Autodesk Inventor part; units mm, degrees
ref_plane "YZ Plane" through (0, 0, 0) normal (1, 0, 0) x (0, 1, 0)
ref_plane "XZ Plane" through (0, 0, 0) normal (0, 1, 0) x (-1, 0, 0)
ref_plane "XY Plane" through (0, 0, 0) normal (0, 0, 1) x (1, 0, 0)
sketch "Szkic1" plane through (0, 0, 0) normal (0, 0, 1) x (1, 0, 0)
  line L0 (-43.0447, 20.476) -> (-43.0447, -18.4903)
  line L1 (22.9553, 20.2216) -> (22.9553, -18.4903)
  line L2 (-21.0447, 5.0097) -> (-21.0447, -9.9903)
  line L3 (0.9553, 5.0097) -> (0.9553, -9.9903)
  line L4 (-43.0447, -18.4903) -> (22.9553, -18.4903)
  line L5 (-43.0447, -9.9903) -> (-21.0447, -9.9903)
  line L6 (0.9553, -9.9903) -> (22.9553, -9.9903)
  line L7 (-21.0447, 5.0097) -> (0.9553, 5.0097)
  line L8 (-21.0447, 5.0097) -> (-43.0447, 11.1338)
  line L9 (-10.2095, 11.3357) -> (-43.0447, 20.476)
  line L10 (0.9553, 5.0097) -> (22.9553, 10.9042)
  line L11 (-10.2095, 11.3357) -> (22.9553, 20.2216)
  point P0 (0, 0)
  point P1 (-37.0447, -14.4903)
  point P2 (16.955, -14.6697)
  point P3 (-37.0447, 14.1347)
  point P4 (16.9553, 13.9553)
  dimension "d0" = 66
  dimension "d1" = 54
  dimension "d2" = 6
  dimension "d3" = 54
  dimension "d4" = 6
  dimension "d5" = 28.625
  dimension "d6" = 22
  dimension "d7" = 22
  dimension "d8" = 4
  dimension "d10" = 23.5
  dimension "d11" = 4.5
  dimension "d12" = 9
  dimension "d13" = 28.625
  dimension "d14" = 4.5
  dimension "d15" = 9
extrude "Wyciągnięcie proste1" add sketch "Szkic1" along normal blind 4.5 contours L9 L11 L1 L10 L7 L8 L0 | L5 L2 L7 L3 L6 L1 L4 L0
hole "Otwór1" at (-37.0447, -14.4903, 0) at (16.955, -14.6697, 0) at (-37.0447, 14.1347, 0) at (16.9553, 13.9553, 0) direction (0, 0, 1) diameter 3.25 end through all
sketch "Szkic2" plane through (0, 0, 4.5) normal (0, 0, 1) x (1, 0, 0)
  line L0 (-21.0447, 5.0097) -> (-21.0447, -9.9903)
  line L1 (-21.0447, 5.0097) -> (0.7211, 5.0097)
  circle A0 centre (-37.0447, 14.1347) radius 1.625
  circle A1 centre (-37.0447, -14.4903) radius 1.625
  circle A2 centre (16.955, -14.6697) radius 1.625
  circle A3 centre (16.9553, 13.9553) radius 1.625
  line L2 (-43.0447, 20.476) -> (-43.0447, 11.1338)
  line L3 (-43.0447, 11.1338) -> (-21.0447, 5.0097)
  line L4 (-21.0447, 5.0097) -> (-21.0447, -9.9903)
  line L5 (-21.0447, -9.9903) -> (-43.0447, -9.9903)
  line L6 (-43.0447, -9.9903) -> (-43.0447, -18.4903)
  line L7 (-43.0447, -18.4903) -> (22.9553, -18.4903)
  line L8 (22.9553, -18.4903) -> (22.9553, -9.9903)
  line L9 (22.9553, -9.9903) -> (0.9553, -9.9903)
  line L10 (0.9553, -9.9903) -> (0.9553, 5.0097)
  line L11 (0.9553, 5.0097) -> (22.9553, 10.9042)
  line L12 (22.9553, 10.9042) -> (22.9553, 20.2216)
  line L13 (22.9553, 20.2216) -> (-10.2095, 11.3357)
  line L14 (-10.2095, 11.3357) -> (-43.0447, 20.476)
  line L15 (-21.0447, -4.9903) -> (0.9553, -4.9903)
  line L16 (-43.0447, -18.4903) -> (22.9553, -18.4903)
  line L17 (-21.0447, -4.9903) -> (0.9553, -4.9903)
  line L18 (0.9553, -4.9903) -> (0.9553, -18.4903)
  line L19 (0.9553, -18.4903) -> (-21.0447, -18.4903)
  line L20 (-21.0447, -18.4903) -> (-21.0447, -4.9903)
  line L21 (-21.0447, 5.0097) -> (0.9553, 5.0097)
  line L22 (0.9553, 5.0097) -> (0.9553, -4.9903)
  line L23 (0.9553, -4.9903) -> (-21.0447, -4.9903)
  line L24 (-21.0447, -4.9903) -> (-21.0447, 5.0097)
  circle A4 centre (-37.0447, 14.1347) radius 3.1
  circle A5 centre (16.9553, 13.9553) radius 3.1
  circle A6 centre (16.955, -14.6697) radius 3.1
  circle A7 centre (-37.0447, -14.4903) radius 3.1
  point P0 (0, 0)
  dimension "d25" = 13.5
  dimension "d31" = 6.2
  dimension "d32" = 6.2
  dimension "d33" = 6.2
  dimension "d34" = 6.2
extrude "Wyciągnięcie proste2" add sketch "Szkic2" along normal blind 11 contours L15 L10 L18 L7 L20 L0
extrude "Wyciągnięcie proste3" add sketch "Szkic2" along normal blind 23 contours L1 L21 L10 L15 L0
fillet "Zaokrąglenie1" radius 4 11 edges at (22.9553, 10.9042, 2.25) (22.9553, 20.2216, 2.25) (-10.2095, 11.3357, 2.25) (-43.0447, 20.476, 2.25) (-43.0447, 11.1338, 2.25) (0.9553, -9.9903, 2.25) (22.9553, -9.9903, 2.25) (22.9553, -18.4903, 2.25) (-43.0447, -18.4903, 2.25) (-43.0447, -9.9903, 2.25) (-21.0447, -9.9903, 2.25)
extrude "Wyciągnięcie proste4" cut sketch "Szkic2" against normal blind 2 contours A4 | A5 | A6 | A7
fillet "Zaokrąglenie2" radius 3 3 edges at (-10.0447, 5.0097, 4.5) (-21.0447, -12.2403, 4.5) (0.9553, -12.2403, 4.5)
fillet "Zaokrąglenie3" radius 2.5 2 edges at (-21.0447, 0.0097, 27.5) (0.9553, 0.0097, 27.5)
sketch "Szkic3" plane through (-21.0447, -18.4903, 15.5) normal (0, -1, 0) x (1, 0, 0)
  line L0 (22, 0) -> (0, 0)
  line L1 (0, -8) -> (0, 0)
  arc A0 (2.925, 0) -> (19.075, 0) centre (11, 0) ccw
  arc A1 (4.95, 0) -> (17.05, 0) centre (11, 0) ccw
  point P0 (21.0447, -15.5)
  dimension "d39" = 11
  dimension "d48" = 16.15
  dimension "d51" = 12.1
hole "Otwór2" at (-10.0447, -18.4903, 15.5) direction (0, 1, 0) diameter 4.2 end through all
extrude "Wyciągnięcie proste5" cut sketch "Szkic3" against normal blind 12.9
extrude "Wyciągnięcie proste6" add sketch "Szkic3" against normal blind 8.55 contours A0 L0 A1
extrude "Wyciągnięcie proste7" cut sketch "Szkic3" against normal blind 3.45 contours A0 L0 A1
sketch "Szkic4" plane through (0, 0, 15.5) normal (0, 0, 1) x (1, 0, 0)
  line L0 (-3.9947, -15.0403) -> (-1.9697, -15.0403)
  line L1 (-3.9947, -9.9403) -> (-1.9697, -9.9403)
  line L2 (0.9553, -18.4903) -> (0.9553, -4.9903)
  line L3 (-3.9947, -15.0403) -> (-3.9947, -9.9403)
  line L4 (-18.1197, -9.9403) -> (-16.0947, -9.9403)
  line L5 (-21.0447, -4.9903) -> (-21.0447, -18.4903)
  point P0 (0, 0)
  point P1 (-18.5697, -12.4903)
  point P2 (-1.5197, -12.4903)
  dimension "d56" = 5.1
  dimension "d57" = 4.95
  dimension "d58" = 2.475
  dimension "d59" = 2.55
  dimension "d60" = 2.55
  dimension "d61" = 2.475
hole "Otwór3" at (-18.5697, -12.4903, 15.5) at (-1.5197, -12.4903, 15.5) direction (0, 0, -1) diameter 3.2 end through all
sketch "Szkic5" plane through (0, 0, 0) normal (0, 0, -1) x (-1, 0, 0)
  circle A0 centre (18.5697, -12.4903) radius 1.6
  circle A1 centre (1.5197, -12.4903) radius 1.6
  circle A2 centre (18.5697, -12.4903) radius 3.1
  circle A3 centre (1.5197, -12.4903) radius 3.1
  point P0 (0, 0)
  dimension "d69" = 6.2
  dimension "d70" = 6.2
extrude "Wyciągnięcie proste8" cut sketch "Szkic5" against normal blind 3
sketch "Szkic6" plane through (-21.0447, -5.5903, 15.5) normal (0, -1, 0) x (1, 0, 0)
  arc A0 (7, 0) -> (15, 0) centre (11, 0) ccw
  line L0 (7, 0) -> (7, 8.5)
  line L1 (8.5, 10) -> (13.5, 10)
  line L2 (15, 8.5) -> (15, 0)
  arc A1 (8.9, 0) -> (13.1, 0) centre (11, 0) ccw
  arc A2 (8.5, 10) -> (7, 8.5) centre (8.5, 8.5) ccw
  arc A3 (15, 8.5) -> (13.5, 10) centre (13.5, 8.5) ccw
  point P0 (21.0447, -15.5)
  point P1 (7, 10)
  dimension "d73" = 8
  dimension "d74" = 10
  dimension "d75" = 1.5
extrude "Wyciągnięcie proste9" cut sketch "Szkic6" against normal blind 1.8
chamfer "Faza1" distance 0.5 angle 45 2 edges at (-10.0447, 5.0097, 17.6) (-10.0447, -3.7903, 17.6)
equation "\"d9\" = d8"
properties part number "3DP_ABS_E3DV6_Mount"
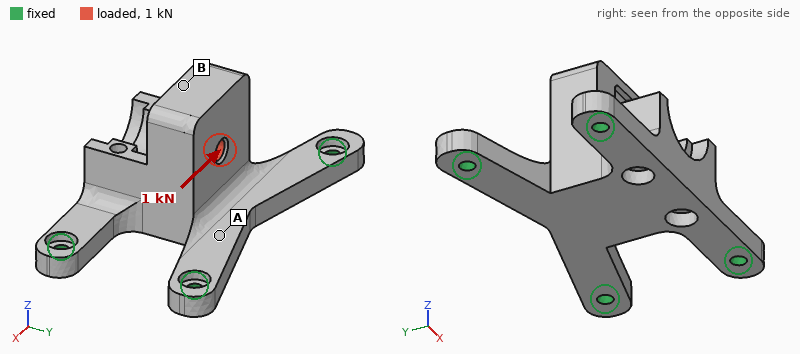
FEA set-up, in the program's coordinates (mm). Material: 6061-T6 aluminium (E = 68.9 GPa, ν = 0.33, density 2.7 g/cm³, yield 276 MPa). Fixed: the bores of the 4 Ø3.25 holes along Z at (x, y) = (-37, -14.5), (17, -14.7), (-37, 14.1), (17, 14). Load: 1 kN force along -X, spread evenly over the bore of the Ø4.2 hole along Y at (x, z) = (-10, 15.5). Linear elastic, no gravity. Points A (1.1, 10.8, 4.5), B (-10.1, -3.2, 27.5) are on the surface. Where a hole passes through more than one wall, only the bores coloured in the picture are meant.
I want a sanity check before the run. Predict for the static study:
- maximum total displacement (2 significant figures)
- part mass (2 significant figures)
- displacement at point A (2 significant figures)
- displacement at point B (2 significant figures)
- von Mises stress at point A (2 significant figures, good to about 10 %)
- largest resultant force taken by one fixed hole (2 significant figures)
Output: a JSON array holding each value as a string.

["47 µm", "35 g", "11 µm", "44 µm", "34 MPa", "340 N"]
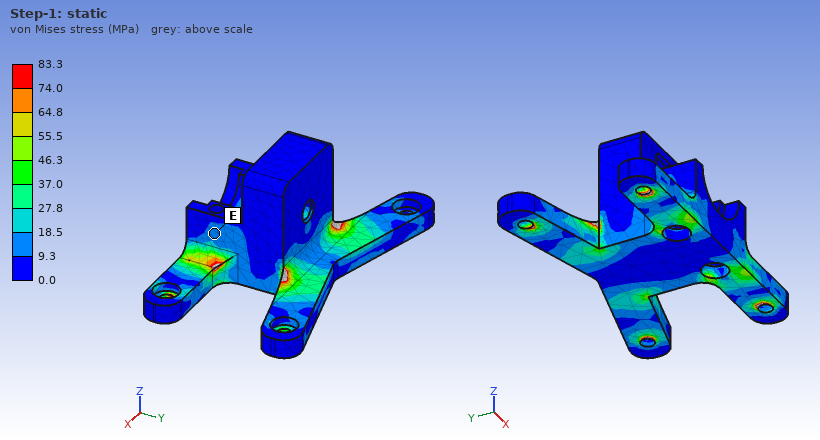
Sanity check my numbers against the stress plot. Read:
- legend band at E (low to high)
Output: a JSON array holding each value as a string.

["9.3 to 18.5 MPa"]
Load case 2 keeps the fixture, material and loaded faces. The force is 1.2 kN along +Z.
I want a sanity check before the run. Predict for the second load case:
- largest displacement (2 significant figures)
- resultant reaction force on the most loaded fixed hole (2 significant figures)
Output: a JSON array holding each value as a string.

["83 µm", "540 N"]
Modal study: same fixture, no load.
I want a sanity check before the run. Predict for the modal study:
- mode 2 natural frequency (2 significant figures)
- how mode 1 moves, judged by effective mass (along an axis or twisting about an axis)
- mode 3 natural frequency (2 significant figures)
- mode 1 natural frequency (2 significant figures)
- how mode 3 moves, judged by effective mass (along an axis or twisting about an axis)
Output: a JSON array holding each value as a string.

["4600 Hz", "along Z", "6600 Hz", "4200 Hz", "along X"]
